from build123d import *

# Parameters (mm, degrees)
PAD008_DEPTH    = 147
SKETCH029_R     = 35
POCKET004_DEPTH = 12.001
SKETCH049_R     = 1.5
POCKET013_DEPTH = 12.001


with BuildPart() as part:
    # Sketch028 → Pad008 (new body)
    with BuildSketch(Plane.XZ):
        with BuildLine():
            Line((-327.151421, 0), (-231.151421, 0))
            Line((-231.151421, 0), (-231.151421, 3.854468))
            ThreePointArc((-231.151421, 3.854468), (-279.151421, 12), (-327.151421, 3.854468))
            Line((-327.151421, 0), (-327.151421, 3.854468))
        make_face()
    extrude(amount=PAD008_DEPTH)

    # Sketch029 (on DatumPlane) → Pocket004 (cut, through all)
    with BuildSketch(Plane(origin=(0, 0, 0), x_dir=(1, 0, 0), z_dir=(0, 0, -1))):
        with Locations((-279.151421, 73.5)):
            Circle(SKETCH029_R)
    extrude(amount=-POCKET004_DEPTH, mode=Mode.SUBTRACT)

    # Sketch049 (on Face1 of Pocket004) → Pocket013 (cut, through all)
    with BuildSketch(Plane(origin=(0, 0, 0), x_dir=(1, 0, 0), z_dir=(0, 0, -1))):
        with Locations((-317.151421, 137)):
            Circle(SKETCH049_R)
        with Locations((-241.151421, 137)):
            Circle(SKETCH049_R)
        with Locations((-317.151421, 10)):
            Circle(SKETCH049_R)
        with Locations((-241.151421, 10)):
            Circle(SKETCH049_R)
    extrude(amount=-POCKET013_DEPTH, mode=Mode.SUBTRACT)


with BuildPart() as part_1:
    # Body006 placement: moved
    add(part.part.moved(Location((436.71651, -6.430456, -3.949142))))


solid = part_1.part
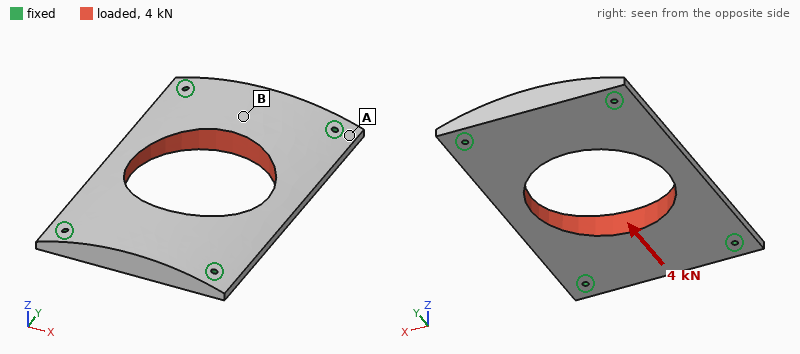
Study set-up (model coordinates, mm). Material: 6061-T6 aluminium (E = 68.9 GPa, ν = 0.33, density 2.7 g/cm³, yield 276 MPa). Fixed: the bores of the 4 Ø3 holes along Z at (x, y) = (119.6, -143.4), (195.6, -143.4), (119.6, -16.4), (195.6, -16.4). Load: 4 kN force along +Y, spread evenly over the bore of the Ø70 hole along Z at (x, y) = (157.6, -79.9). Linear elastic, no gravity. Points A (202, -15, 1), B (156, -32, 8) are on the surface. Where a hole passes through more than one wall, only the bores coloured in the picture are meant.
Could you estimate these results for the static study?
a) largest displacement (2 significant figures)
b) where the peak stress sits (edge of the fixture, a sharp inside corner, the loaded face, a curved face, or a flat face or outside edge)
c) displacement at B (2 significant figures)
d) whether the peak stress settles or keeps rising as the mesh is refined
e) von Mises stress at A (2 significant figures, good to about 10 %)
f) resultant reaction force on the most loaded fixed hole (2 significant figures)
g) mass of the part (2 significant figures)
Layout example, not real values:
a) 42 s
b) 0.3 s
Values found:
a) 5.4 µm
b) edge of the fixture
c) 4.8 µm
d) keeps rising
e) 4.7 MPa
f) 1.0 kN
g) 240 g
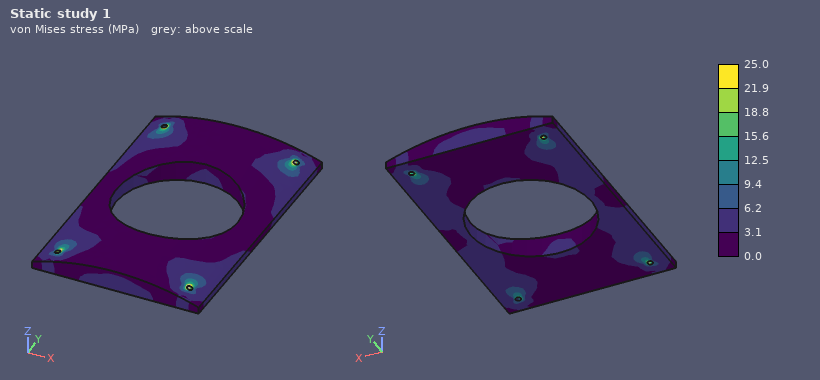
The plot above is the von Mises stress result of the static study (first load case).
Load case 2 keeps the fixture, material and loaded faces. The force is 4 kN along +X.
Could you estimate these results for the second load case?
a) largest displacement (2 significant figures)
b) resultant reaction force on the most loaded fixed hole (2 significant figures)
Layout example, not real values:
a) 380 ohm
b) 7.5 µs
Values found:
a) 18 µm
b) 1.2 kN
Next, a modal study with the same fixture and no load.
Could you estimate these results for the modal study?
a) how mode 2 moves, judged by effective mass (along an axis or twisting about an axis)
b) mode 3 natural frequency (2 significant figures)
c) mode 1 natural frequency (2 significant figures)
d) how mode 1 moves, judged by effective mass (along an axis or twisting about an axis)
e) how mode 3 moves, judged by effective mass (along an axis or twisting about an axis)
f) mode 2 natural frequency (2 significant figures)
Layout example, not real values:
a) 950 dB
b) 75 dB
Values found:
a) twisting about Y
b) 4100 Hz
c) 2100 Hz
d) along Z
e) twisting about X
f) 3500 Hz
